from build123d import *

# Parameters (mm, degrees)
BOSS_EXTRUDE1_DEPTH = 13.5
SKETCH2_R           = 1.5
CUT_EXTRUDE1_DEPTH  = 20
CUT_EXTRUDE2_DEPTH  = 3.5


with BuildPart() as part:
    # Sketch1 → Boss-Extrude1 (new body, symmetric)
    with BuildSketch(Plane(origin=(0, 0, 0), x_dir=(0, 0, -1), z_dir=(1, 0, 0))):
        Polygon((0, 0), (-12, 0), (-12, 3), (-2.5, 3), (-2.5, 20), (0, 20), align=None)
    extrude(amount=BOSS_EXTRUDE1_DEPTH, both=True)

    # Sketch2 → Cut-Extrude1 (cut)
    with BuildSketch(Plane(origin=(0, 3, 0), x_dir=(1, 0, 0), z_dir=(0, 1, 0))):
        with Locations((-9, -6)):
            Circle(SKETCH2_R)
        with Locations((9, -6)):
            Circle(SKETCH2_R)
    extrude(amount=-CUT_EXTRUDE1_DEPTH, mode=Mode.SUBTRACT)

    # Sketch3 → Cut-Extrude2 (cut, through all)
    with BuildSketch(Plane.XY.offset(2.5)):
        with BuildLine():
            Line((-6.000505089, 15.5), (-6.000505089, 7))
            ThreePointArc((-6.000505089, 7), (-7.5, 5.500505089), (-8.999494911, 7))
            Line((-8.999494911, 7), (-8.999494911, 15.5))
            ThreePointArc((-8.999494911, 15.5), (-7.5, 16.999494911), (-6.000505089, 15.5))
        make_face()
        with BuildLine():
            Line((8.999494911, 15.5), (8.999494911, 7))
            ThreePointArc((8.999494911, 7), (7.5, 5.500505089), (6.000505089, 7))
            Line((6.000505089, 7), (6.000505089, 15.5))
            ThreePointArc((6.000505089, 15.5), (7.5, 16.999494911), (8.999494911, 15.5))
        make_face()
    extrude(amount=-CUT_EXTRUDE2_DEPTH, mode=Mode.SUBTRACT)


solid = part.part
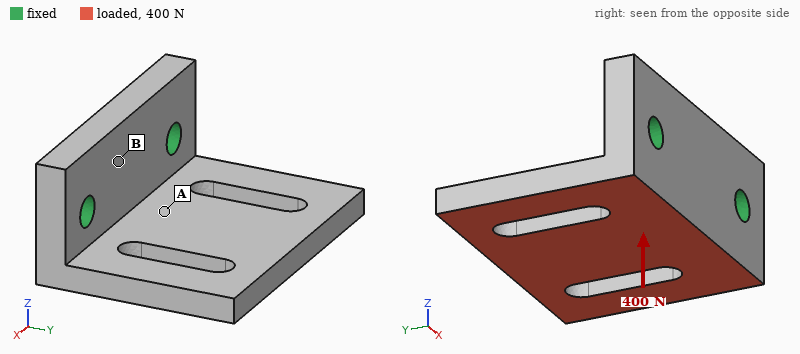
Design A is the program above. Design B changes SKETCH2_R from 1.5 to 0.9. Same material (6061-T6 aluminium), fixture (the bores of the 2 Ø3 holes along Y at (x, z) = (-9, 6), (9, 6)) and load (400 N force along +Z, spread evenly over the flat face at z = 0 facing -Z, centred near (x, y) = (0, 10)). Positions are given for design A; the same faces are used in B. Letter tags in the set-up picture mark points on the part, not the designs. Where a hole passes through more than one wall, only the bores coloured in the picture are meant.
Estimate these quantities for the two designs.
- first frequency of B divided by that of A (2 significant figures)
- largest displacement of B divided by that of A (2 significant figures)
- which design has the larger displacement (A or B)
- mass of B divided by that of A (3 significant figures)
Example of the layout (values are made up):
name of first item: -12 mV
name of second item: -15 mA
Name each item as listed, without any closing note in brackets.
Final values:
first frequency of B divided by that of A: 0.95
largest displacement of B divided by that of A: 1.1
which design has the larger displacement: B
mass of B divided by that of A: 1.01
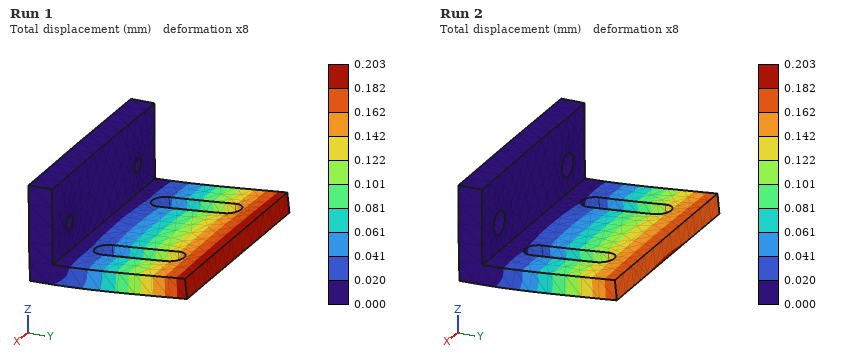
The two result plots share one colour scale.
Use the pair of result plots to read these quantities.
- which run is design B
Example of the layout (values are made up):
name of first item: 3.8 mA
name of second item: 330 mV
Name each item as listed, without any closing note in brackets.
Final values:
which run is design B: Run 1
